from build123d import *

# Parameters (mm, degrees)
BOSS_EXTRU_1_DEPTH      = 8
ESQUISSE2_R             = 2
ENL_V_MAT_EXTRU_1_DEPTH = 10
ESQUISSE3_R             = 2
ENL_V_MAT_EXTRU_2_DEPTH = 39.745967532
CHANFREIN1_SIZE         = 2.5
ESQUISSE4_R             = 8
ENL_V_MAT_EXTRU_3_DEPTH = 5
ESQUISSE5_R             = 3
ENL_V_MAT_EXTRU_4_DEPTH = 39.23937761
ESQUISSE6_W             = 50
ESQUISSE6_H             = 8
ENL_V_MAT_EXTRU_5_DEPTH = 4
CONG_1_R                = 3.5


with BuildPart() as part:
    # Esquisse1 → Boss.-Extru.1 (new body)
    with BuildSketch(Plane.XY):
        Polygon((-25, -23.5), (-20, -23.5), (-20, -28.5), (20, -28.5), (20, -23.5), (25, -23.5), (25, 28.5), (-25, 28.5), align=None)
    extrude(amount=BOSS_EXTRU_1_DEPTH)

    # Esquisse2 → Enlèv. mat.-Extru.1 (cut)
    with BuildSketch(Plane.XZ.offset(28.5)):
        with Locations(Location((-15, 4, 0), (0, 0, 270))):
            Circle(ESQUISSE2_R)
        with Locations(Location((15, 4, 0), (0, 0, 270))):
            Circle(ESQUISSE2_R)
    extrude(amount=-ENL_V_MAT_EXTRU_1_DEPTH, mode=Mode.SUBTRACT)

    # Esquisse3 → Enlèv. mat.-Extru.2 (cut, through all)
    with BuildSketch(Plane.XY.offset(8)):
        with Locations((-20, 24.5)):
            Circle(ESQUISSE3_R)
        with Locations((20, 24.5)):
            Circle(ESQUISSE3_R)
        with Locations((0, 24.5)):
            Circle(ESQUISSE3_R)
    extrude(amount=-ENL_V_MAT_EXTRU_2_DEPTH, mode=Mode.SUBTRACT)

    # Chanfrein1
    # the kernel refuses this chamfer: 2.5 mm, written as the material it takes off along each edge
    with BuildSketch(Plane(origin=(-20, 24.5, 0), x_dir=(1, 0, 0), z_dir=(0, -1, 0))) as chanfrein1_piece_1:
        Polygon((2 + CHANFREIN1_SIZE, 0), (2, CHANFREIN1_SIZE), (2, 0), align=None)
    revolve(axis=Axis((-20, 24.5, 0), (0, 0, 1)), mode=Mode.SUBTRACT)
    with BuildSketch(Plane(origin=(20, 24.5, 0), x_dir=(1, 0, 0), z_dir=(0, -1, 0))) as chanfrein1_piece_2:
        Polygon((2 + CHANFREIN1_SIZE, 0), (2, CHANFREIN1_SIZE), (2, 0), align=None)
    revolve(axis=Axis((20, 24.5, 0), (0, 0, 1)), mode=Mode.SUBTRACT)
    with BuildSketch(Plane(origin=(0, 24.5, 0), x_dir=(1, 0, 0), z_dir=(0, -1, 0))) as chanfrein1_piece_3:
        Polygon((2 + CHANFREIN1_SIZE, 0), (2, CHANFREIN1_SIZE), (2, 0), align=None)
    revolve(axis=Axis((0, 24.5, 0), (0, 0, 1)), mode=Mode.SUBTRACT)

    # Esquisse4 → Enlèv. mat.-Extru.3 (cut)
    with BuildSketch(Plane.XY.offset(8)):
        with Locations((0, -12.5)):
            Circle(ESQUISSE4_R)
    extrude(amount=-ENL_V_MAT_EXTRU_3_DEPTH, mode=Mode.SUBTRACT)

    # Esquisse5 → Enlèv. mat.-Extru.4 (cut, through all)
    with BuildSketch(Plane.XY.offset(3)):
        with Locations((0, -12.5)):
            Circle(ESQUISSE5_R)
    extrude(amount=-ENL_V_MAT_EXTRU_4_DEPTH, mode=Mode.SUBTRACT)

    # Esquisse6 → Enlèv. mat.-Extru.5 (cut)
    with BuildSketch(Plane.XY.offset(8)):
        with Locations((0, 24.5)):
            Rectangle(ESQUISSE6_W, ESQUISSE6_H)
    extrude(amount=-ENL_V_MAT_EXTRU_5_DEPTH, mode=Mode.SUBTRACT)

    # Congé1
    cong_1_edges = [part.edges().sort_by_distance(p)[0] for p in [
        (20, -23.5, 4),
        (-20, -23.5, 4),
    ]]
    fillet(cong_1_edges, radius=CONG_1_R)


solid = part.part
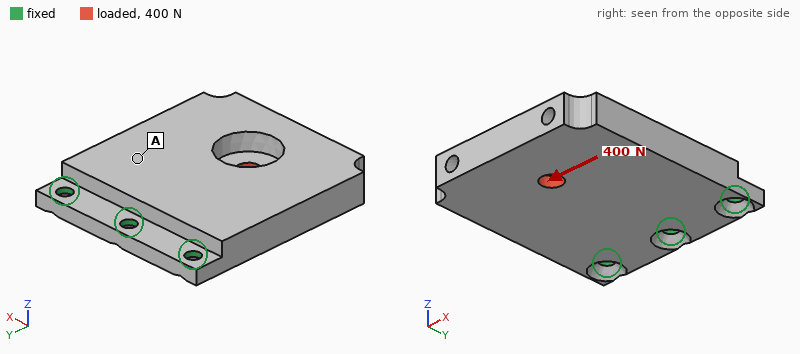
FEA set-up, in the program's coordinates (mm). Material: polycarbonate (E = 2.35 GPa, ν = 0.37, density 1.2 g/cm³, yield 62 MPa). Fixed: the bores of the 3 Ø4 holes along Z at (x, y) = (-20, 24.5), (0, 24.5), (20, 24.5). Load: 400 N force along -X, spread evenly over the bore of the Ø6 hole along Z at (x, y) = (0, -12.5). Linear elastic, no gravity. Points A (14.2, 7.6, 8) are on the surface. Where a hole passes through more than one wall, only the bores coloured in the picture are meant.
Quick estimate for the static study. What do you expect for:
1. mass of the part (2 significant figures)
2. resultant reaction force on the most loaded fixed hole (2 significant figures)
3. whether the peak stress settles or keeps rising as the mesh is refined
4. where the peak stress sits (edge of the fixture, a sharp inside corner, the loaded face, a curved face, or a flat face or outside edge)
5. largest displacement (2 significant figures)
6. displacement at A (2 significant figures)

23 g
380 N
keeps rising
edge of the fixture
0.28 mm
0.079 mm
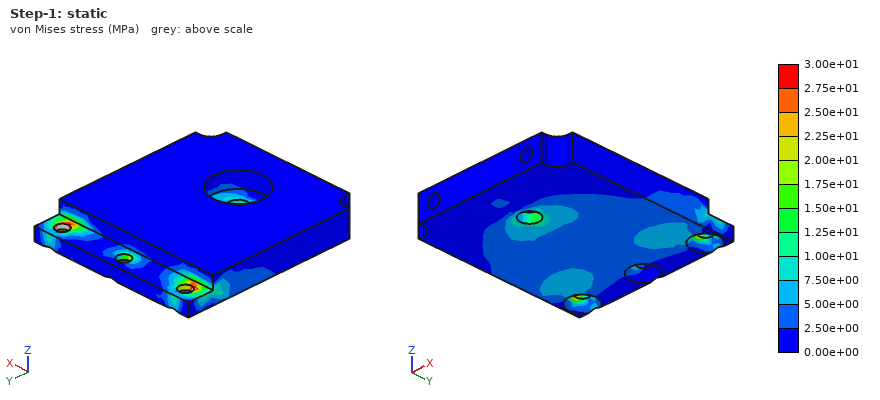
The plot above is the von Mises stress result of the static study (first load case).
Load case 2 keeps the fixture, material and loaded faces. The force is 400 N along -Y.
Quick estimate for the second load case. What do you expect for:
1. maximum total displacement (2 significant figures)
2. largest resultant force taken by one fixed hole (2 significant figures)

0.78 mm
150 N
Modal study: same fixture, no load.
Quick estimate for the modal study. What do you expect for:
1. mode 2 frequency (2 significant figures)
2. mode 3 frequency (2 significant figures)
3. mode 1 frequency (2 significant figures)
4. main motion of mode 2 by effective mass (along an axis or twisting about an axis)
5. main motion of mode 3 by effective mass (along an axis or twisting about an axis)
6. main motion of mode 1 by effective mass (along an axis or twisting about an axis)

1200 Hz
2100 Hz
250 Hz
twisting about Y
along X
along Z
